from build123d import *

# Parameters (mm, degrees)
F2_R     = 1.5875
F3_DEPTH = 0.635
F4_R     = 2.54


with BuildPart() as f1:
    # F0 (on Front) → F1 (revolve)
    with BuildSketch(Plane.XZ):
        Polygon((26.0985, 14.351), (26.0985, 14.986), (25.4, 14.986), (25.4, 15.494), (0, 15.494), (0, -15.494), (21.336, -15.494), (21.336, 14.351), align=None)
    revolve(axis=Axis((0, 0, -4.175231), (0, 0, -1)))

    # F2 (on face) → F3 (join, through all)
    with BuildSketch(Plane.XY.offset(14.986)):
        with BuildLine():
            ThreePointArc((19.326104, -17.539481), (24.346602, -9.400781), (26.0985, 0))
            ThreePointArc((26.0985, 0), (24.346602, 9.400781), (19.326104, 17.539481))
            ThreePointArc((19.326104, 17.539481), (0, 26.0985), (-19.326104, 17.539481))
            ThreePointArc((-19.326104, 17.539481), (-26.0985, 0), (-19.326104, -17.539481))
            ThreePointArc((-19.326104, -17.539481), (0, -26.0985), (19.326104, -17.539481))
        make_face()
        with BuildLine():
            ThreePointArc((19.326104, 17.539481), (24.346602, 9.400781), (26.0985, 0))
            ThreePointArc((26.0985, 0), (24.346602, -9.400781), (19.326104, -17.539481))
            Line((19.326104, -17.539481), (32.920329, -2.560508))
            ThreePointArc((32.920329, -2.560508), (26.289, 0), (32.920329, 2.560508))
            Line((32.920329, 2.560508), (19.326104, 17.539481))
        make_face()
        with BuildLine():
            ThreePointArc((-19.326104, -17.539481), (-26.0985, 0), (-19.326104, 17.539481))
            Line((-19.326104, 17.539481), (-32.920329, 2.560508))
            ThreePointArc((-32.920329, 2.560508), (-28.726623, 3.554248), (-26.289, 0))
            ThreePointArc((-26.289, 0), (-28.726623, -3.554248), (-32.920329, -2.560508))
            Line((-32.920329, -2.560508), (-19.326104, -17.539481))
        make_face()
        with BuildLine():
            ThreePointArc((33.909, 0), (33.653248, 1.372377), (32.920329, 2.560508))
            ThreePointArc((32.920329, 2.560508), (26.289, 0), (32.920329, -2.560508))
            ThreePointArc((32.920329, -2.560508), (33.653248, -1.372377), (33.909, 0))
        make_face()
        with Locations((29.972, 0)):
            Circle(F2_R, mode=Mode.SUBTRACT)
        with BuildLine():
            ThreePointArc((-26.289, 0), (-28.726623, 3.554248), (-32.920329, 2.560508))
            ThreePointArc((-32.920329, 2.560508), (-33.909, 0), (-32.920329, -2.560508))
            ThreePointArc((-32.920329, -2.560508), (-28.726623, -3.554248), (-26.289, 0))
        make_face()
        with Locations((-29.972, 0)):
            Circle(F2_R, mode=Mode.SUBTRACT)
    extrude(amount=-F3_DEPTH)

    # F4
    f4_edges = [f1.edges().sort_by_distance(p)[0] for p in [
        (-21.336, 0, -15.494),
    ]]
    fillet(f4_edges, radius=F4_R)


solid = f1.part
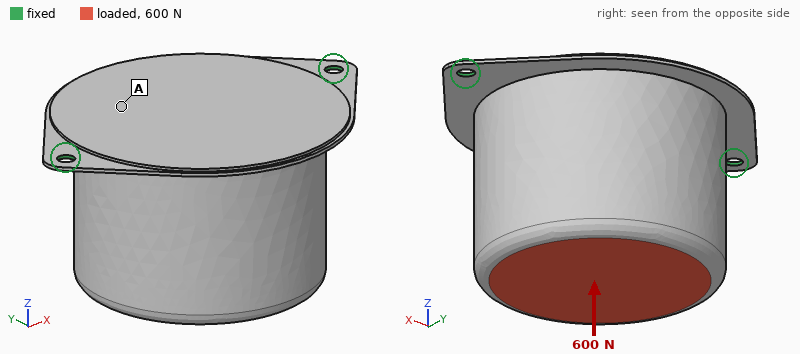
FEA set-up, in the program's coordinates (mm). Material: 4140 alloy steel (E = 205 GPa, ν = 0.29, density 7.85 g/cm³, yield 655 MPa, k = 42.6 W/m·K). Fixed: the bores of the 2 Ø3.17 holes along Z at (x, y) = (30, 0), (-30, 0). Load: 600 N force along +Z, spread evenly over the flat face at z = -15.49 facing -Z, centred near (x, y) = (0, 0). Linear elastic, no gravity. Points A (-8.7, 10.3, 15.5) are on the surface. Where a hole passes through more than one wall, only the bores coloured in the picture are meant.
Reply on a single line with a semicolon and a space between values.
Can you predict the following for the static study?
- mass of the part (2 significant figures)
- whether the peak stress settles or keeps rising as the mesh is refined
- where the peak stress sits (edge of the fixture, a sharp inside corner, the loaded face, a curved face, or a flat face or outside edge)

350 g; keeps rising; edge of the fixture
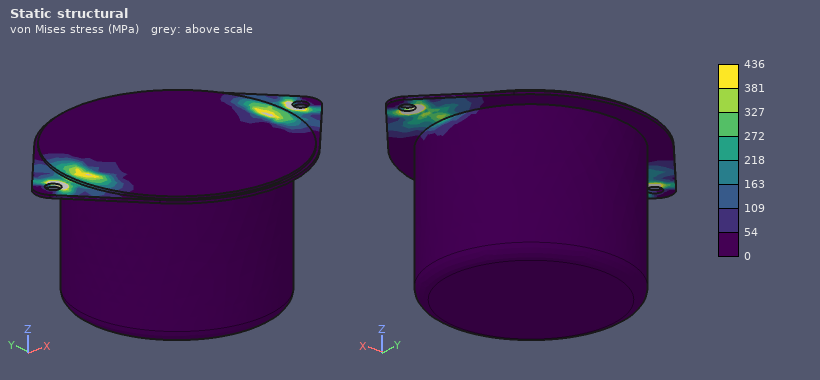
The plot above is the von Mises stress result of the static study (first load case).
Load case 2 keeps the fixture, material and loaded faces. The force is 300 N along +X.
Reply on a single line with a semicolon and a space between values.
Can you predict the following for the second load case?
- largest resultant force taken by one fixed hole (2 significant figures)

230 N
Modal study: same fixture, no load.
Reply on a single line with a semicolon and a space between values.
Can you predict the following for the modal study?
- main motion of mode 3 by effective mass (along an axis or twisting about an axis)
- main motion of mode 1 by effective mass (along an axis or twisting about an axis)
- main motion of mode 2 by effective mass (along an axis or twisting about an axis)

along X; along Y; along Z
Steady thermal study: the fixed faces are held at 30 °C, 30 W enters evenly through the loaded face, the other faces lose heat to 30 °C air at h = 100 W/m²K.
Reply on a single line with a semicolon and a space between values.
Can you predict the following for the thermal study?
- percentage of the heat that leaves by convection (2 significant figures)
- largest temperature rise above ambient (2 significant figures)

90 %; 48 K
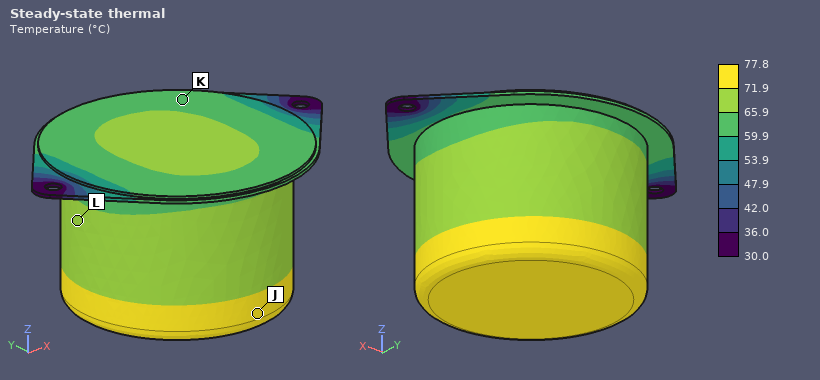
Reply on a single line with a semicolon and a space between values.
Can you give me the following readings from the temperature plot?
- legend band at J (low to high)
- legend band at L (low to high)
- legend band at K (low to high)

71.9 to 77.8 °C; 65.9 to 71.9 °C; 59.9 to 65.9 °C
